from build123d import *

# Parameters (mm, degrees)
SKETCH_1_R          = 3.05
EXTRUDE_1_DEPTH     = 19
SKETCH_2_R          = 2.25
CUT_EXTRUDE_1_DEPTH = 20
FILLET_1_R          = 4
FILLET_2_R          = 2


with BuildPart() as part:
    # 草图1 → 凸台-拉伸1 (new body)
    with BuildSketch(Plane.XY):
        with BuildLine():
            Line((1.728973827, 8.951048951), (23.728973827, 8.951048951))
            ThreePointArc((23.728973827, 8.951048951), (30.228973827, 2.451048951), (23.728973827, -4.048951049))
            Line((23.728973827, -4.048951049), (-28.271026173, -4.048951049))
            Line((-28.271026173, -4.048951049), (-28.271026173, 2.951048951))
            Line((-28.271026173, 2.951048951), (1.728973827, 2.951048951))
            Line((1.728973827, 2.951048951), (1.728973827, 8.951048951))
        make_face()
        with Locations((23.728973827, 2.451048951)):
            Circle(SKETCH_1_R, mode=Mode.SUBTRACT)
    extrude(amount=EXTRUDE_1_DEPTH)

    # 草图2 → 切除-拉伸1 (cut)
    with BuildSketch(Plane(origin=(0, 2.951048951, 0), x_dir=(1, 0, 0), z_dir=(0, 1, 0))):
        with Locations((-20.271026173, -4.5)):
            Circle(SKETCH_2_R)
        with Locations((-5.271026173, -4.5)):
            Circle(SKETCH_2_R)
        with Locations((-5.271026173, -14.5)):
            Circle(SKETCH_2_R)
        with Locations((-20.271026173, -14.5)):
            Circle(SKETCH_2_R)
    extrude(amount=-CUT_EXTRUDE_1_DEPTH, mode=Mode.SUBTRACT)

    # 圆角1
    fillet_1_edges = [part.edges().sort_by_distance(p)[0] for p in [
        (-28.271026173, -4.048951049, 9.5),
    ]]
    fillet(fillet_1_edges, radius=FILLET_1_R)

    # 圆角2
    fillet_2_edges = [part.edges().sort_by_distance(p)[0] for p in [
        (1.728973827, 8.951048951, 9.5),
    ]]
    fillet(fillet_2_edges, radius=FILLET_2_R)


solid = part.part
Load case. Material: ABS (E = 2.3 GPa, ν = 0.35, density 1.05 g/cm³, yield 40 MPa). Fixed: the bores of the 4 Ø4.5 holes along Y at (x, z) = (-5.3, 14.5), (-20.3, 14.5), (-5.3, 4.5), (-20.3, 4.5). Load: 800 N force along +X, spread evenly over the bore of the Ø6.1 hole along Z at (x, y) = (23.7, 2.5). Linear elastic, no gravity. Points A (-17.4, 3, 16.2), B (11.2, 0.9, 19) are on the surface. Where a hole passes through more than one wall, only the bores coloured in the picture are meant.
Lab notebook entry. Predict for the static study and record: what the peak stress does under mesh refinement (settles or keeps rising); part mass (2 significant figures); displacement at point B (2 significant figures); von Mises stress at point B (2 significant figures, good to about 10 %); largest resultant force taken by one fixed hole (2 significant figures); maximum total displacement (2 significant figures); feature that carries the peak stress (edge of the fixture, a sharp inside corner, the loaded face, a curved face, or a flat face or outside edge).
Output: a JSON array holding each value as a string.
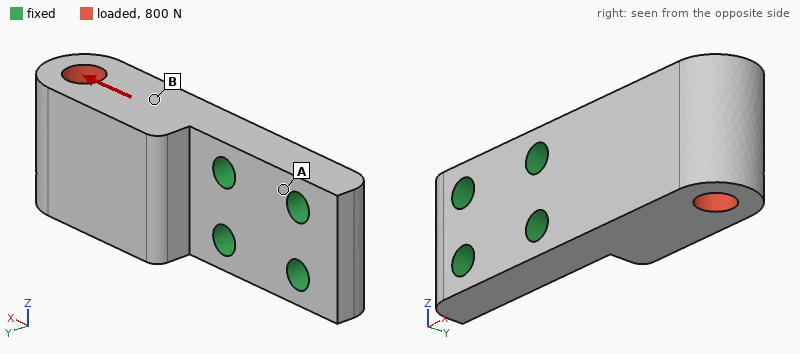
["keeps rising", "10 g", "0.18 mm", "3.9 MPa", "390 N", "0.49 mm", "edge of the fixture"]
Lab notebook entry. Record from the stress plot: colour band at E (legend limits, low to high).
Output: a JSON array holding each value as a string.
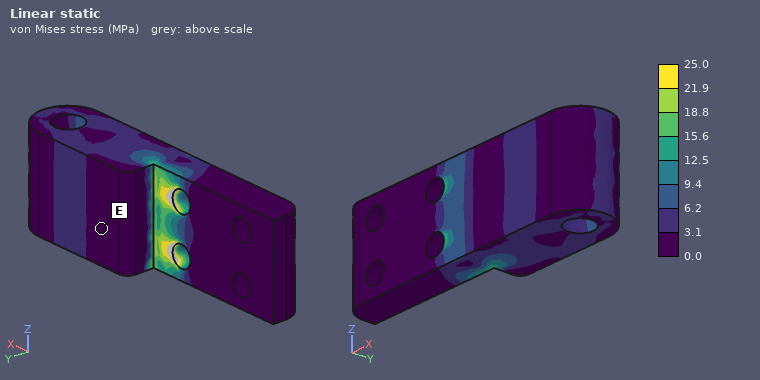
["0.0 to 3.1 MPa"]
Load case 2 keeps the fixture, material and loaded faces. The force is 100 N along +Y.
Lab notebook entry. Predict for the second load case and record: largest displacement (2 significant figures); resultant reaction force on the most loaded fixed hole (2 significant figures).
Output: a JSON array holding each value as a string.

["0.55 mm", "56 N"]
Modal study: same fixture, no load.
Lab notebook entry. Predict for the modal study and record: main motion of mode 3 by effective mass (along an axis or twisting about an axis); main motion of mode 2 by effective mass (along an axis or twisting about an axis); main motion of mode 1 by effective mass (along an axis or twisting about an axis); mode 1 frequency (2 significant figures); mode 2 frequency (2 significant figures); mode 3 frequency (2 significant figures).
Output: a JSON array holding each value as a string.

["twisting about X", "along Z", "along Y", "1300 Hz", "2800 Hz", "4500 Hz"]
